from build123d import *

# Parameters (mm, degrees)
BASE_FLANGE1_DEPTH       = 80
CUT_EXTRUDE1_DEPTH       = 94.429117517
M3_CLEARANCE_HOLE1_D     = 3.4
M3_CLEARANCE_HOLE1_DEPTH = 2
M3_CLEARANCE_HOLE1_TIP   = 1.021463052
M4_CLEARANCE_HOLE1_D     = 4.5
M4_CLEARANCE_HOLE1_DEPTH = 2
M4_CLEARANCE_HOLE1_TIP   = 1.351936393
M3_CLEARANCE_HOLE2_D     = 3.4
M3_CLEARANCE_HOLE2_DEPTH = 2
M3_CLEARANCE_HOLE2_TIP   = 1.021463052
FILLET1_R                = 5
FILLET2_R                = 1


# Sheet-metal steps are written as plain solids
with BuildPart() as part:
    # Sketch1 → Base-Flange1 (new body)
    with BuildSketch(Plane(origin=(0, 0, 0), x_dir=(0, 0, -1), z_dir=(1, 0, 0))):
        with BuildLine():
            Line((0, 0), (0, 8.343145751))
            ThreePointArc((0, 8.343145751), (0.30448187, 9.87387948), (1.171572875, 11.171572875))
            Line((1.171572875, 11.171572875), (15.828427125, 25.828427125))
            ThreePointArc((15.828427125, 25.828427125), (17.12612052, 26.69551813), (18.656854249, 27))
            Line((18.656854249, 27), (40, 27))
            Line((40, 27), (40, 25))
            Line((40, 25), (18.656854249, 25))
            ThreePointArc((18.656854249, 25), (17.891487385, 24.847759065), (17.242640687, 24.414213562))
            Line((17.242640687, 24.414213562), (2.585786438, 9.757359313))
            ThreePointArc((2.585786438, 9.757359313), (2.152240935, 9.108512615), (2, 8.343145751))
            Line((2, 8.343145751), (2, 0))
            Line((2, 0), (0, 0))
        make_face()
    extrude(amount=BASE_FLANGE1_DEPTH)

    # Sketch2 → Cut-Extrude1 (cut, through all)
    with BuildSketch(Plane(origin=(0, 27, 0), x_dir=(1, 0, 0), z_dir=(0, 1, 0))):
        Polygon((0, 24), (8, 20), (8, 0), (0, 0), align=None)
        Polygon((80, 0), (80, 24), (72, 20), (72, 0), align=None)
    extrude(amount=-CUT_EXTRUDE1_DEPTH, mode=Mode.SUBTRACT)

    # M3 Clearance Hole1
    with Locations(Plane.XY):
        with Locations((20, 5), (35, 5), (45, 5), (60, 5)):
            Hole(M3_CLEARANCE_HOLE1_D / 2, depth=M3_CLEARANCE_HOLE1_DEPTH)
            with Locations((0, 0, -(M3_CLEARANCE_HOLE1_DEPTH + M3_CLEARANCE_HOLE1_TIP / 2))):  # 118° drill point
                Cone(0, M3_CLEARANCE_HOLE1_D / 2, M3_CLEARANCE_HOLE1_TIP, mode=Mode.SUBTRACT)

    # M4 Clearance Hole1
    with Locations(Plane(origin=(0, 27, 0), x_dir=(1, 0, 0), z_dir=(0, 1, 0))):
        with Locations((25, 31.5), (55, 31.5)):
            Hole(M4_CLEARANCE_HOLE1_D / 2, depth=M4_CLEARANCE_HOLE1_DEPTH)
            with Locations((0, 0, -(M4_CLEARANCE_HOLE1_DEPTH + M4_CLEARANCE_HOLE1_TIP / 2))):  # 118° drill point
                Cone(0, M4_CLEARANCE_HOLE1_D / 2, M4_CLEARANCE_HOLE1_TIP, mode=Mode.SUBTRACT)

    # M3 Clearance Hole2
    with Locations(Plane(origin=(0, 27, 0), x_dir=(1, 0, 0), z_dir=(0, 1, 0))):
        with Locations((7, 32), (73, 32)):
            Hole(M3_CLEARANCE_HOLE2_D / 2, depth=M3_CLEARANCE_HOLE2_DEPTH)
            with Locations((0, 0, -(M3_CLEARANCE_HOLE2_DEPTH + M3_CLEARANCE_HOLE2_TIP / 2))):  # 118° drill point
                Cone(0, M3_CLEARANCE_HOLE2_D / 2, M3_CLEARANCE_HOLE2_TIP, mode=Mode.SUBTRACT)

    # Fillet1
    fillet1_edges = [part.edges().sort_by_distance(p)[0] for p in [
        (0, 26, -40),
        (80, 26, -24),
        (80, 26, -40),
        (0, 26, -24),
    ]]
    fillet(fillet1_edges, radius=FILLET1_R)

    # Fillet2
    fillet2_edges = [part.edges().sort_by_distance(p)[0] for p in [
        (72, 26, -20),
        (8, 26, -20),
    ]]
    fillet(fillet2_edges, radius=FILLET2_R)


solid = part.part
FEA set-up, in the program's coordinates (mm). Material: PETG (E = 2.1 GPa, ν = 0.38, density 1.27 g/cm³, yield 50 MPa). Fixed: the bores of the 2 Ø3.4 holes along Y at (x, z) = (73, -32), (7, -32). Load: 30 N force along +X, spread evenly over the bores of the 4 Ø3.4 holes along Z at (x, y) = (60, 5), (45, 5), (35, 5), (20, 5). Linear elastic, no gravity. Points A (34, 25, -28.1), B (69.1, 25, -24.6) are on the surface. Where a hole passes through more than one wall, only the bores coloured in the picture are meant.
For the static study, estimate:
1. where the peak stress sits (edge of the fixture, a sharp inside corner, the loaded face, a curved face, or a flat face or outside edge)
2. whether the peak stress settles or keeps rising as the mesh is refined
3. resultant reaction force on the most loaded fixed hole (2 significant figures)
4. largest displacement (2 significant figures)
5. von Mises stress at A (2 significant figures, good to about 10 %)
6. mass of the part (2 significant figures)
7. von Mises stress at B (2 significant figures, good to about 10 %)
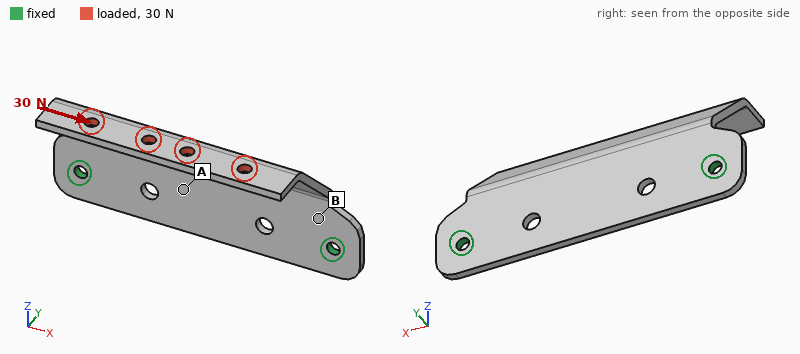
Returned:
edge of the fixture
keeps rising
23 N
1.1 mm
1.9 MPa
9.4 g
4.3 MPa
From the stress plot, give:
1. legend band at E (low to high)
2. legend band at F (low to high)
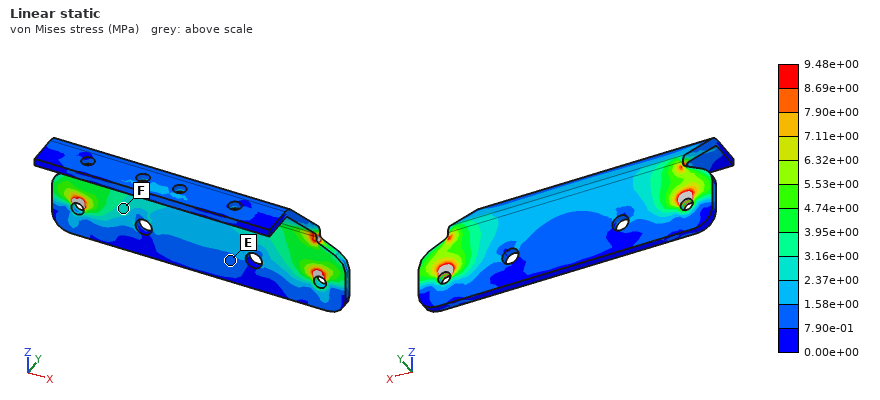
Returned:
7.90e-01 to 1.58e+00 MPa
2.37e+00 to 3.16e+00 MPa
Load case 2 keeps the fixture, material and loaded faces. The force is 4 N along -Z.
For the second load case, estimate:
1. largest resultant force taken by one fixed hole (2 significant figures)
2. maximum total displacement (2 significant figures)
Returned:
2.8 N
0.92 mm
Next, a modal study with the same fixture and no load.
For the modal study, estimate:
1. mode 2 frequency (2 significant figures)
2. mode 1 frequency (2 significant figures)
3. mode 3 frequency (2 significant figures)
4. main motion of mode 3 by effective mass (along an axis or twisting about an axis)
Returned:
400 Hz
180 Hz
710 Hz
along Y
